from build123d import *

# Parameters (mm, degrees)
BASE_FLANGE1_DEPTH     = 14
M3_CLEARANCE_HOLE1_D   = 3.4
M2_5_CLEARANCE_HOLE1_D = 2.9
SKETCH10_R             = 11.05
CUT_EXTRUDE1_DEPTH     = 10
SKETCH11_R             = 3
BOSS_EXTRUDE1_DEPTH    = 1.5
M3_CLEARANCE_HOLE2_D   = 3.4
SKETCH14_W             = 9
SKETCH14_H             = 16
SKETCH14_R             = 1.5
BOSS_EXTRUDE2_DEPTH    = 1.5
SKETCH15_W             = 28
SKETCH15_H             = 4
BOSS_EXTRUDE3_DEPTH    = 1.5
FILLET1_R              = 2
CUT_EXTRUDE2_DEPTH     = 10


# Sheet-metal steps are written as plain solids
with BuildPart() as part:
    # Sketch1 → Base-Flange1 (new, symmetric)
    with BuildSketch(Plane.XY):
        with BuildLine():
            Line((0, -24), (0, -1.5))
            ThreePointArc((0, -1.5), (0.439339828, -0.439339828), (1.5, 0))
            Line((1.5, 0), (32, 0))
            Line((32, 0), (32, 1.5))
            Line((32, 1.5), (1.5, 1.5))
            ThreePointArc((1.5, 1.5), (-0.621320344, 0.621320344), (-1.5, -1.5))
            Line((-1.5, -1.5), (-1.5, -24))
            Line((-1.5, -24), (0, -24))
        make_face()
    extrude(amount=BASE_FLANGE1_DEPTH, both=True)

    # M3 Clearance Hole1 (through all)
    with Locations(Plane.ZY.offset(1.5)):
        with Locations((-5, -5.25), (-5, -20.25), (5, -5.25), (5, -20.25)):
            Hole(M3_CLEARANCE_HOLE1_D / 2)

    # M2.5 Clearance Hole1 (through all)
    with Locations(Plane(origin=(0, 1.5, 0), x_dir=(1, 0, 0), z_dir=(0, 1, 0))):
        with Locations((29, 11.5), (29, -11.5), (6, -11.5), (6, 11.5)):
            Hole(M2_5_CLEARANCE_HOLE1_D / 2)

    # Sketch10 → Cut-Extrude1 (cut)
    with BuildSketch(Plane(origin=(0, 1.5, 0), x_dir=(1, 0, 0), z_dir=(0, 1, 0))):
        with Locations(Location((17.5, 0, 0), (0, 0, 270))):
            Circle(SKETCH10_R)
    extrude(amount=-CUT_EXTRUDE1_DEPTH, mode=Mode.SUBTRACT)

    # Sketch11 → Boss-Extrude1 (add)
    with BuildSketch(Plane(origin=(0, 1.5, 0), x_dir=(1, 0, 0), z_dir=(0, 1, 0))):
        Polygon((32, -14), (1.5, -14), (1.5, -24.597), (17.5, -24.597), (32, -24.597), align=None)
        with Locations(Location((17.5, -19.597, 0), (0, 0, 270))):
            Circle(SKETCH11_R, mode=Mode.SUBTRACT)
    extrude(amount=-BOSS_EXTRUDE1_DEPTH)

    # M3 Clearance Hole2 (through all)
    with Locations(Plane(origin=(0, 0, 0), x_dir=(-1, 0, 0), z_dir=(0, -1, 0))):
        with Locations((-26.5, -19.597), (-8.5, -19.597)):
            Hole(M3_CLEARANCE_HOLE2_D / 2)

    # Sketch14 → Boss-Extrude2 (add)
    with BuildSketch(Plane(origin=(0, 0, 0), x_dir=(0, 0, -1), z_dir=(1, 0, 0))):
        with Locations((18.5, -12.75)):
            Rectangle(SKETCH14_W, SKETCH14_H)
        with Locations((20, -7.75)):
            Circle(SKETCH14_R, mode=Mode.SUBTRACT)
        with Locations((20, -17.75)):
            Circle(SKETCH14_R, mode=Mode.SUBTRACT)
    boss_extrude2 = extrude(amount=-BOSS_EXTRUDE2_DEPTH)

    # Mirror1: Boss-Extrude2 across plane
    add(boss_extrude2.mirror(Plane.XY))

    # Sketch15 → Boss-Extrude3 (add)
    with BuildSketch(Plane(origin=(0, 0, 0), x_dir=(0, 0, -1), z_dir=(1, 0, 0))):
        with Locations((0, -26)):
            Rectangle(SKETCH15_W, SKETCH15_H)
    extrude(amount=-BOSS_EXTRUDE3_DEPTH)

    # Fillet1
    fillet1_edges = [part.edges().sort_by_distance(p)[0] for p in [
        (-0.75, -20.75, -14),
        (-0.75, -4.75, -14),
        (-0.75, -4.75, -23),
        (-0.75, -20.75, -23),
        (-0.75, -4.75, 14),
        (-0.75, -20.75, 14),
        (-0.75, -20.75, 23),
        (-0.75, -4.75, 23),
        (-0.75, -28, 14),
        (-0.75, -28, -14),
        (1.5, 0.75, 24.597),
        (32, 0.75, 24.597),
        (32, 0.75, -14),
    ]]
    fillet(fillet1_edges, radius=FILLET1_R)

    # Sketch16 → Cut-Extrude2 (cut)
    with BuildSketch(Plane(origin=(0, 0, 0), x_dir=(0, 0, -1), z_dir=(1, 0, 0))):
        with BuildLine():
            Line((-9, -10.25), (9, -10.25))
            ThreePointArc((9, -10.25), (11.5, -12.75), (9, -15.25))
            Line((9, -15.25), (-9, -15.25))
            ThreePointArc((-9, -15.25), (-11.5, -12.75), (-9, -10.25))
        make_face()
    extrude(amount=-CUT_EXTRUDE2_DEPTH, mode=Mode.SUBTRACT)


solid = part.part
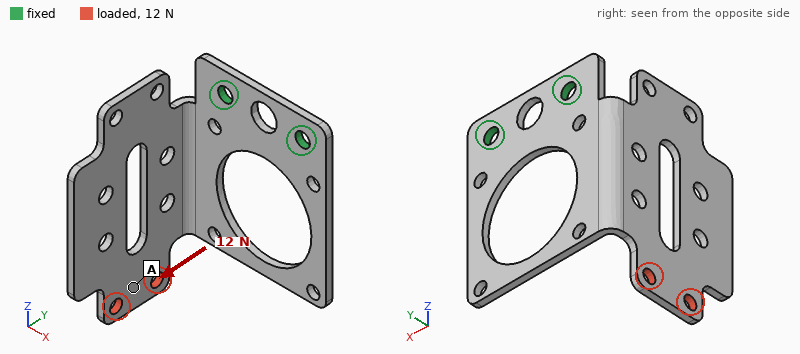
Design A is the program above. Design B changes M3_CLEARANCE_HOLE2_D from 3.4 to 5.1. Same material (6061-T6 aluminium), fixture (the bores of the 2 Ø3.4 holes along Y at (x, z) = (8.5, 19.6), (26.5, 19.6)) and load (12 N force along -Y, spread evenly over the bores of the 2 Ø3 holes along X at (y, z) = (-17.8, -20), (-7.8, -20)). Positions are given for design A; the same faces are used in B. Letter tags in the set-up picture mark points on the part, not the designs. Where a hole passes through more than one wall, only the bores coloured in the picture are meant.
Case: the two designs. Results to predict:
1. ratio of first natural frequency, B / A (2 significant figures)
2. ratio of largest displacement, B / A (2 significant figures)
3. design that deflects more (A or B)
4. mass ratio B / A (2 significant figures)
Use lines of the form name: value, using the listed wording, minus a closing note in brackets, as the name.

ratio of first natural frequency, B / A: 1.0
ratio of largest displacement, B / A: 0.92
design that deflects more: A
mass ratio B / A: 0.99
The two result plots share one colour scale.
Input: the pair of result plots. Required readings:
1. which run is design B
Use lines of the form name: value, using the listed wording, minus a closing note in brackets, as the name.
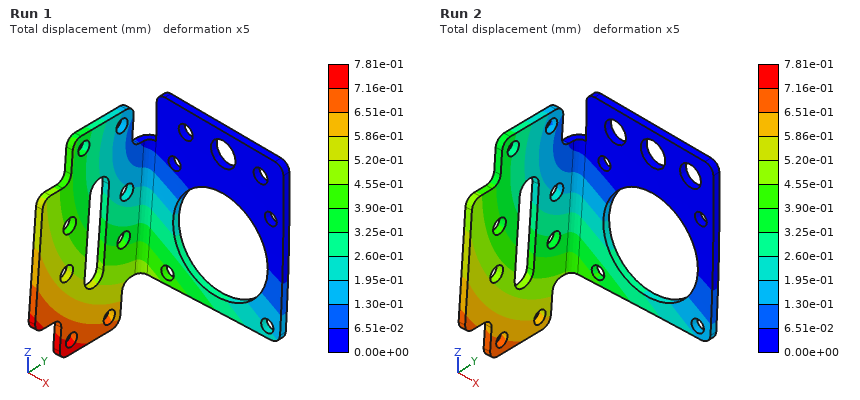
which run is design B: Run 2
